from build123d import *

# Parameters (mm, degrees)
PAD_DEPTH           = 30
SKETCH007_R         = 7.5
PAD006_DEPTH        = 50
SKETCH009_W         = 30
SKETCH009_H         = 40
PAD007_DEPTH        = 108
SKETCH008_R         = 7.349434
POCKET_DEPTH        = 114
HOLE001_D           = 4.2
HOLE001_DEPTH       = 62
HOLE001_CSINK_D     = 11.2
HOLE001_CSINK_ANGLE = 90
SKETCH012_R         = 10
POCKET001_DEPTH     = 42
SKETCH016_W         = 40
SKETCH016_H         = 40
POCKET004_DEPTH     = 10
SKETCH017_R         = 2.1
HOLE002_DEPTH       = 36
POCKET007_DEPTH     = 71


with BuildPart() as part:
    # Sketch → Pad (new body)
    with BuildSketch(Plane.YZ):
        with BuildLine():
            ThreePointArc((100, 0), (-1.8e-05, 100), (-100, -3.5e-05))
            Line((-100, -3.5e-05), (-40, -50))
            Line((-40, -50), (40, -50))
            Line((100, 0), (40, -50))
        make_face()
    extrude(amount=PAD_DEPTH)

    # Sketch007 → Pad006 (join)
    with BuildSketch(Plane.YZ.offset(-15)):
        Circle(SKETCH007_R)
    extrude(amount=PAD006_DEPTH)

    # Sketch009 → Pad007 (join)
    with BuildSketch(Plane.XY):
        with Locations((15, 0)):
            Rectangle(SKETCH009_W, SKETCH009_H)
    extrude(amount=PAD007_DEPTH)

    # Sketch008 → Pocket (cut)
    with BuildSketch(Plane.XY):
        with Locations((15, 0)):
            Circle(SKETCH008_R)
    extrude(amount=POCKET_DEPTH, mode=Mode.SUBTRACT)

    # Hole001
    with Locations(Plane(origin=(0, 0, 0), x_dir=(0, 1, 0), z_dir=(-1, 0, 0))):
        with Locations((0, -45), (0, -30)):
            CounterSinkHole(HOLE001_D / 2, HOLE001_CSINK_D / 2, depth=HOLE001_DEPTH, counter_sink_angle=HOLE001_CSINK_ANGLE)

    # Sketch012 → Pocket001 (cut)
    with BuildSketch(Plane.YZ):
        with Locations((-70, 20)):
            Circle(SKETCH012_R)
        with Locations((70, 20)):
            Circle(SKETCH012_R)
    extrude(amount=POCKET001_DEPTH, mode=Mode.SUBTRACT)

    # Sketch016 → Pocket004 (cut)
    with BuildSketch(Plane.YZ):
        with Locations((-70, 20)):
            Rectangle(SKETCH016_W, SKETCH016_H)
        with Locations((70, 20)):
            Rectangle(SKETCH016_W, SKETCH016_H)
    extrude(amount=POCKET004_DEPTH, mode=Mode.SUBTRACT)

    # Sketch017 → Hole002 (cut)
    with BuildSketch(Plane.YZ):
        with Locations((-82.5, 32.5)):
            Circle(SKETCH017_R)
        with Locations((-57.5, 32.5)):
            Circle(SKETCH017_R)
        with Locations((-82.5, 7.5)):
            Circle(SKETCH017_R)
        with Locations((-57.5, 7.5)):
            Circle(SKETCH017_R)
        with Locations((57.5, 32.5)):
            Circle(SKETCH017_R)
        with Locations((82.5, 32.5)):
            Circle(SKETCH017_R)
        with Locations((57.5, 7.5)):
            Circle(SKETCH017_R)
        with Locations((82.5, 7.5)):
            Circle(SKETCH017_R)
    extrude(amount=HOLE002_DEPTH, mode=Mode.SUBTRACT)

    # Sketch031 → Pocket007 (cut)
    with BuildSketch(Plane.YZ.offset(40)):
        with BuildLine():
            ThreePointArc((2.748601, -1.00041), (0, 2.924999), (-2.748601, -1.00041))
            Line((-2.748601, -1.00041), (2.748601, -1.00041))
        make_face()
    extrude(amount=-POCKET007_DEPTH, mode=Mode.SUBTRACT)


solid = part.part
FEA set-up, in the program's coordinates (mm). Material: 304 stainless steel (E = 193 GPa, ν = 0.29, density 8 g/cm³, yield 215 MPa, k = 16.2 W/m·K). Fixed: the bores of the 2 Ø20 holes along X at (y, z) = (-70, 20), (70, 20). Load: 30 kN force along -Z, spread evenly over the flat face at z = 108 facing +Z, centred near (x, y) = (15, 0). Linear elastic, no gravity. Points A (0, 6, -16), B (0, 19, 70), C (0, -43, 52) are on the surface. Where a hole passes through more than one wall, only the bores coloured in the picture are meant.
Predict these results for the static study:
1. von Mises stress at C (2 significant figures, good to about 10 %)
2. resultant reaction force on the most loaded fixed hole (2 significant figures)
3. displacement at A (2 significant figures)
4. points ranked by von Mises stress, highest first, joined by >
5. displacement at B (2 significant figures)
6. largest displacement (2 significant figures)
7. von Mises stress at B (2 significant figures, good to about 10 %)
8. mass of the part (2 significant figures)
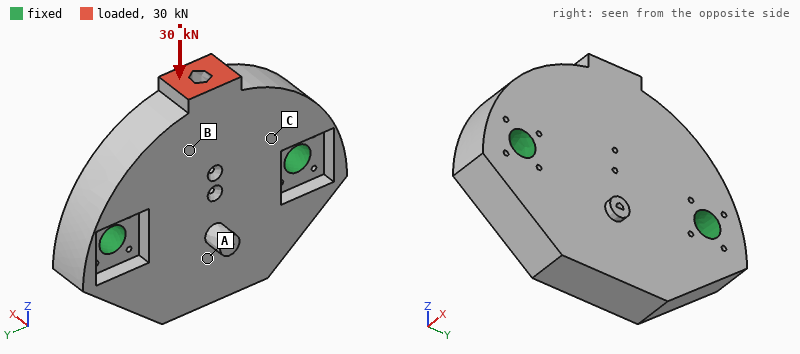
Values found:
7.9 MPa
15 kN
5.8 µm
B > C > A
9.7 µm
17 µm
15 MPa
5.0 kg
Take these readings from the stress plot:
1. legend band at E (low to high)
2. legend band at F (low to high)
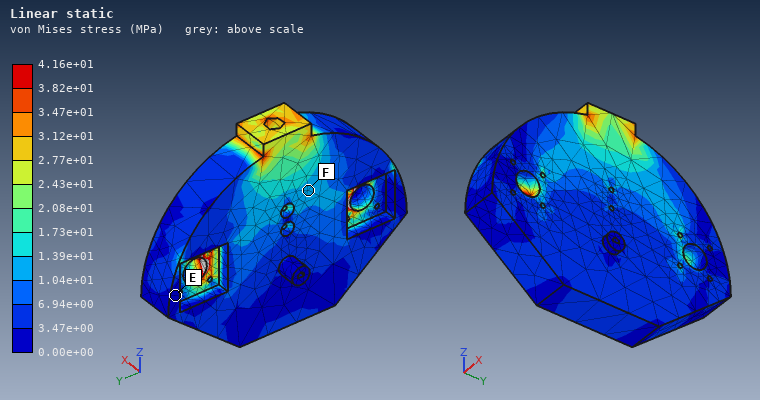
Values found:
0.00e+00 to 3.47e+00 MPa
1.04e+01 to 1.39e+01 MPa
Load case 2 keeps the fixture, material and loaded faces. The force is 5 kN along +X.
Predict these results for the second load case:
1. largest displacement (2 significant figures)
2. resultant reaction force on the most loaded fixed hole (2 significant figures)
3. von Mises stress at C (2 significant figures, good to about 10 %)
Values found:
49 µm
3.0 kN
14 MPa
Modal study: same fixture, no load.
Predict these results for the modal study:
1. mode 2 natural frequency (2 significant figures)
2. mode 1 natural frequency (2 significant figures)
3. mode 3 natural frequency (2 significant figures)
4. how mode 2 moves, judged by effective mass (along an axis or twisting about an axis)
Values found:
3300 Hz
2200 Hz
6400 Hz
along X
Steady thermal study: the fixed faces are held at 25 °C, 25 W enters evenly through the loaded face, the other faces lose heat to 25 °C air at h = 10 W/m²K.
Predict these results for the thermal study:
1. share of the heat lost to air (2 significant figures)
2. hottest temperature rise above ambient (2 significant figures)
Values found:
31 %
62 K
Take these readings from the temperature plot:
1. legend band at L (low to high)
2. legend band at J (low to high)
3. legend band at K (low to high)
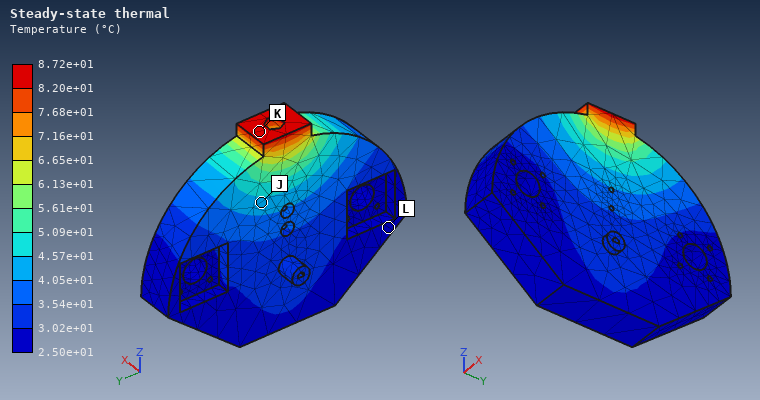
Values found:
2.50e+01 to 3.02e+01 °C
4.05e+01 to 4.57e+01 °C
8.20e+01 to 8.72e+01 °C
